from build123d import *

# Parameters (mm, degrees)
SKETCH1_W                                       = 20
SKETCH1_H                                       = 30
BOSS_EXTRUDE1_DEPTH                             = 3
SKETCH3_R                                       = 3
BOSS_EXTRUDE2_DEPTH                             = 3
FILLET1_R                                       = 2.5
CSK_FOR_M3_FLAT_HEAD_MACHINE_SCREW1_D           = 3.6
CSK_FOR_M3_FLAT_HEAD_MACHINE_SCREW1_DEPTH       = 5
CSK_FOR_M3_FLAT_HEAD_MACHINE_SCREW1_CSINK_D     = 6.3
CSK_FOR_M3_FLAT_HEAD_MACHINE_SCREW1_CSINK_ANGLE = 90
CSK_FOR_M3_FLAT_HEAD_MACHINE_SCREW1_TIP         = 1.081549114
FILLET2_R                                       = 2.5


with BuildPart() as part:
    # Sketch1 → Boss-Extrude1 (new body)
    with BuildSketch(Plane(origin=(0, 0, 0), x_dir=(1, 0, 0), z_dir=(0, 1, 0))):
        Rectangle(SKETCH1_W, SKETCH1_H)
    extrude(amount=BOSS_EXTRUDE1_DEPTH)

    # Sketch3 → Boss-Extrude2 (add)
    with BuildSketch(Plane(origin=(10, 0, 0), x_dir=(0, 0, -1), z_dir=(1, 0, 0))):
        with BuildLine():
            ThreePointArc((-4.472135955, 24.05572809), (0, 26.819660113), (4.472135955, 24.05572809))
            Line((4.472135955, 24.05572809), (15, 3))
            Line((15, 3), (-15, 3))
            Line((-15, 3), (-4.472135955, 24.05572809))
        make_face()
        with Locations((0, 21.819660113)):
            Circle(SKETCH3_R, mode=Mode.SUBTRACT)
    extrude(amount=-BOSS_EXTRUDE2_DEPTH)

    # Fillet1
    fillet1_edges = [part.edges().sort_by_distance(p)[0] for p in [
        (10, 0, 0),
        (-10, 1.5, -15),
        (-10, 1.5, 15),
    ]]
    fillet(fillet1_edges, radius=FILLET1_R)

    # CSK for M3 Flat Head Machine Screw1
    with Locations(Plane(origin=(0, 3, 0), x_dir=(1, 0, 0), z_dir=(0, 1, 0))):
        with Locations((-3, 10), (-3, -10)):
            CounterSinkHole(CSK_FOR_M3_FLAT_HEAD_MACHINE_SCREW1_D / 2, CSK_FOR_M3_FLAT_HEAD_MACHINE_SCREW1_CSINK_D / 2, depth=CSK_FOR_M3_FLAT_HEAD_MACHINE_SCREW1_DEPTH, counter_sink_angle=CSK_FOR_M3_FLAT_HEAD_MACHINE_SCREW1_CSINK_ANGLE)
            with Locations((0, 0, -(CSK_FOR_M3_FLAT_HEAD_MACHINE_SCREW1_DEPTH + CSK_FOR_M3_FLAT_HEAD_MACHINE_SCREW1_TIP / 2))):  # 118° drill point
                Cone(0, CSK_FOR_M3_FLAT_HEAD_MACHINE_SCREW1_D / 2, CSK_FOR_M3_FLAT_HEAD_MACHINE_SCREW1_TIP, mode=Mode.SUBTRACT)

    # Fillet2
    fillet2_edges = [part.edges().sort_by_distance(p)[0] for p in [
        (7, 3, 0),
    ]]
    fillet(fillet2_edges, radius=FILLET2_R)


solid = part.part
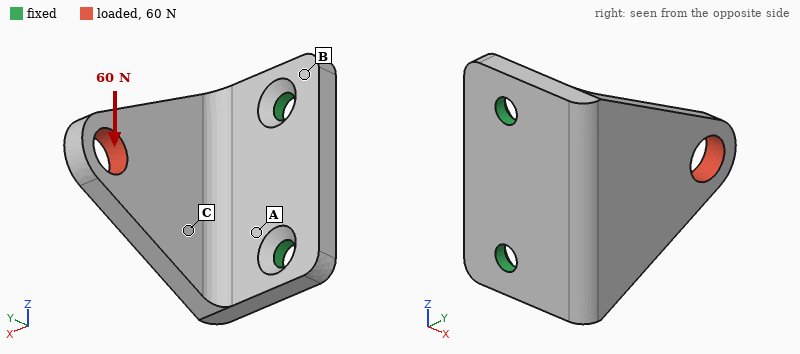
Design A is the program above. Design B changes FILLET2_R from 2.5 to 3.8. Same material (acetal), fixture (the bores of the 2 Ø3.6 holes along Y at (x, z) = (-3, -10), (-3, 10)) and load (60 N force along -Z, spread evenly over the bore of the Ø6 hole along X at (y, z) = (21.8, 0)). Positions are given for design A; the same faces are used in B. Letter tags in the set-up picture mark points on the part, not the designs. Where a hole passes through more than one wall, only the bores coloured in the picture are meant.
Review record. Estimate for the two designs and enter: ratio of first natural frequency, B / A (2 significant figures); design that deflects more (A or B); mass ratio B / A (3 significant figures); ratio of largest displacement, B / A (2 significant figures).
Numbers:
1.0
A
1.02
0.89
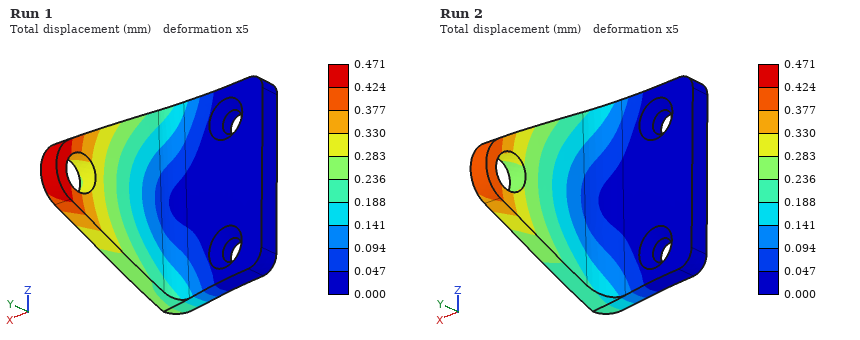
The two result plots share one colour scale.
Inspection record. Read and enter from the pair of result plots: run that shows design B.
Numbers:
Run 2
